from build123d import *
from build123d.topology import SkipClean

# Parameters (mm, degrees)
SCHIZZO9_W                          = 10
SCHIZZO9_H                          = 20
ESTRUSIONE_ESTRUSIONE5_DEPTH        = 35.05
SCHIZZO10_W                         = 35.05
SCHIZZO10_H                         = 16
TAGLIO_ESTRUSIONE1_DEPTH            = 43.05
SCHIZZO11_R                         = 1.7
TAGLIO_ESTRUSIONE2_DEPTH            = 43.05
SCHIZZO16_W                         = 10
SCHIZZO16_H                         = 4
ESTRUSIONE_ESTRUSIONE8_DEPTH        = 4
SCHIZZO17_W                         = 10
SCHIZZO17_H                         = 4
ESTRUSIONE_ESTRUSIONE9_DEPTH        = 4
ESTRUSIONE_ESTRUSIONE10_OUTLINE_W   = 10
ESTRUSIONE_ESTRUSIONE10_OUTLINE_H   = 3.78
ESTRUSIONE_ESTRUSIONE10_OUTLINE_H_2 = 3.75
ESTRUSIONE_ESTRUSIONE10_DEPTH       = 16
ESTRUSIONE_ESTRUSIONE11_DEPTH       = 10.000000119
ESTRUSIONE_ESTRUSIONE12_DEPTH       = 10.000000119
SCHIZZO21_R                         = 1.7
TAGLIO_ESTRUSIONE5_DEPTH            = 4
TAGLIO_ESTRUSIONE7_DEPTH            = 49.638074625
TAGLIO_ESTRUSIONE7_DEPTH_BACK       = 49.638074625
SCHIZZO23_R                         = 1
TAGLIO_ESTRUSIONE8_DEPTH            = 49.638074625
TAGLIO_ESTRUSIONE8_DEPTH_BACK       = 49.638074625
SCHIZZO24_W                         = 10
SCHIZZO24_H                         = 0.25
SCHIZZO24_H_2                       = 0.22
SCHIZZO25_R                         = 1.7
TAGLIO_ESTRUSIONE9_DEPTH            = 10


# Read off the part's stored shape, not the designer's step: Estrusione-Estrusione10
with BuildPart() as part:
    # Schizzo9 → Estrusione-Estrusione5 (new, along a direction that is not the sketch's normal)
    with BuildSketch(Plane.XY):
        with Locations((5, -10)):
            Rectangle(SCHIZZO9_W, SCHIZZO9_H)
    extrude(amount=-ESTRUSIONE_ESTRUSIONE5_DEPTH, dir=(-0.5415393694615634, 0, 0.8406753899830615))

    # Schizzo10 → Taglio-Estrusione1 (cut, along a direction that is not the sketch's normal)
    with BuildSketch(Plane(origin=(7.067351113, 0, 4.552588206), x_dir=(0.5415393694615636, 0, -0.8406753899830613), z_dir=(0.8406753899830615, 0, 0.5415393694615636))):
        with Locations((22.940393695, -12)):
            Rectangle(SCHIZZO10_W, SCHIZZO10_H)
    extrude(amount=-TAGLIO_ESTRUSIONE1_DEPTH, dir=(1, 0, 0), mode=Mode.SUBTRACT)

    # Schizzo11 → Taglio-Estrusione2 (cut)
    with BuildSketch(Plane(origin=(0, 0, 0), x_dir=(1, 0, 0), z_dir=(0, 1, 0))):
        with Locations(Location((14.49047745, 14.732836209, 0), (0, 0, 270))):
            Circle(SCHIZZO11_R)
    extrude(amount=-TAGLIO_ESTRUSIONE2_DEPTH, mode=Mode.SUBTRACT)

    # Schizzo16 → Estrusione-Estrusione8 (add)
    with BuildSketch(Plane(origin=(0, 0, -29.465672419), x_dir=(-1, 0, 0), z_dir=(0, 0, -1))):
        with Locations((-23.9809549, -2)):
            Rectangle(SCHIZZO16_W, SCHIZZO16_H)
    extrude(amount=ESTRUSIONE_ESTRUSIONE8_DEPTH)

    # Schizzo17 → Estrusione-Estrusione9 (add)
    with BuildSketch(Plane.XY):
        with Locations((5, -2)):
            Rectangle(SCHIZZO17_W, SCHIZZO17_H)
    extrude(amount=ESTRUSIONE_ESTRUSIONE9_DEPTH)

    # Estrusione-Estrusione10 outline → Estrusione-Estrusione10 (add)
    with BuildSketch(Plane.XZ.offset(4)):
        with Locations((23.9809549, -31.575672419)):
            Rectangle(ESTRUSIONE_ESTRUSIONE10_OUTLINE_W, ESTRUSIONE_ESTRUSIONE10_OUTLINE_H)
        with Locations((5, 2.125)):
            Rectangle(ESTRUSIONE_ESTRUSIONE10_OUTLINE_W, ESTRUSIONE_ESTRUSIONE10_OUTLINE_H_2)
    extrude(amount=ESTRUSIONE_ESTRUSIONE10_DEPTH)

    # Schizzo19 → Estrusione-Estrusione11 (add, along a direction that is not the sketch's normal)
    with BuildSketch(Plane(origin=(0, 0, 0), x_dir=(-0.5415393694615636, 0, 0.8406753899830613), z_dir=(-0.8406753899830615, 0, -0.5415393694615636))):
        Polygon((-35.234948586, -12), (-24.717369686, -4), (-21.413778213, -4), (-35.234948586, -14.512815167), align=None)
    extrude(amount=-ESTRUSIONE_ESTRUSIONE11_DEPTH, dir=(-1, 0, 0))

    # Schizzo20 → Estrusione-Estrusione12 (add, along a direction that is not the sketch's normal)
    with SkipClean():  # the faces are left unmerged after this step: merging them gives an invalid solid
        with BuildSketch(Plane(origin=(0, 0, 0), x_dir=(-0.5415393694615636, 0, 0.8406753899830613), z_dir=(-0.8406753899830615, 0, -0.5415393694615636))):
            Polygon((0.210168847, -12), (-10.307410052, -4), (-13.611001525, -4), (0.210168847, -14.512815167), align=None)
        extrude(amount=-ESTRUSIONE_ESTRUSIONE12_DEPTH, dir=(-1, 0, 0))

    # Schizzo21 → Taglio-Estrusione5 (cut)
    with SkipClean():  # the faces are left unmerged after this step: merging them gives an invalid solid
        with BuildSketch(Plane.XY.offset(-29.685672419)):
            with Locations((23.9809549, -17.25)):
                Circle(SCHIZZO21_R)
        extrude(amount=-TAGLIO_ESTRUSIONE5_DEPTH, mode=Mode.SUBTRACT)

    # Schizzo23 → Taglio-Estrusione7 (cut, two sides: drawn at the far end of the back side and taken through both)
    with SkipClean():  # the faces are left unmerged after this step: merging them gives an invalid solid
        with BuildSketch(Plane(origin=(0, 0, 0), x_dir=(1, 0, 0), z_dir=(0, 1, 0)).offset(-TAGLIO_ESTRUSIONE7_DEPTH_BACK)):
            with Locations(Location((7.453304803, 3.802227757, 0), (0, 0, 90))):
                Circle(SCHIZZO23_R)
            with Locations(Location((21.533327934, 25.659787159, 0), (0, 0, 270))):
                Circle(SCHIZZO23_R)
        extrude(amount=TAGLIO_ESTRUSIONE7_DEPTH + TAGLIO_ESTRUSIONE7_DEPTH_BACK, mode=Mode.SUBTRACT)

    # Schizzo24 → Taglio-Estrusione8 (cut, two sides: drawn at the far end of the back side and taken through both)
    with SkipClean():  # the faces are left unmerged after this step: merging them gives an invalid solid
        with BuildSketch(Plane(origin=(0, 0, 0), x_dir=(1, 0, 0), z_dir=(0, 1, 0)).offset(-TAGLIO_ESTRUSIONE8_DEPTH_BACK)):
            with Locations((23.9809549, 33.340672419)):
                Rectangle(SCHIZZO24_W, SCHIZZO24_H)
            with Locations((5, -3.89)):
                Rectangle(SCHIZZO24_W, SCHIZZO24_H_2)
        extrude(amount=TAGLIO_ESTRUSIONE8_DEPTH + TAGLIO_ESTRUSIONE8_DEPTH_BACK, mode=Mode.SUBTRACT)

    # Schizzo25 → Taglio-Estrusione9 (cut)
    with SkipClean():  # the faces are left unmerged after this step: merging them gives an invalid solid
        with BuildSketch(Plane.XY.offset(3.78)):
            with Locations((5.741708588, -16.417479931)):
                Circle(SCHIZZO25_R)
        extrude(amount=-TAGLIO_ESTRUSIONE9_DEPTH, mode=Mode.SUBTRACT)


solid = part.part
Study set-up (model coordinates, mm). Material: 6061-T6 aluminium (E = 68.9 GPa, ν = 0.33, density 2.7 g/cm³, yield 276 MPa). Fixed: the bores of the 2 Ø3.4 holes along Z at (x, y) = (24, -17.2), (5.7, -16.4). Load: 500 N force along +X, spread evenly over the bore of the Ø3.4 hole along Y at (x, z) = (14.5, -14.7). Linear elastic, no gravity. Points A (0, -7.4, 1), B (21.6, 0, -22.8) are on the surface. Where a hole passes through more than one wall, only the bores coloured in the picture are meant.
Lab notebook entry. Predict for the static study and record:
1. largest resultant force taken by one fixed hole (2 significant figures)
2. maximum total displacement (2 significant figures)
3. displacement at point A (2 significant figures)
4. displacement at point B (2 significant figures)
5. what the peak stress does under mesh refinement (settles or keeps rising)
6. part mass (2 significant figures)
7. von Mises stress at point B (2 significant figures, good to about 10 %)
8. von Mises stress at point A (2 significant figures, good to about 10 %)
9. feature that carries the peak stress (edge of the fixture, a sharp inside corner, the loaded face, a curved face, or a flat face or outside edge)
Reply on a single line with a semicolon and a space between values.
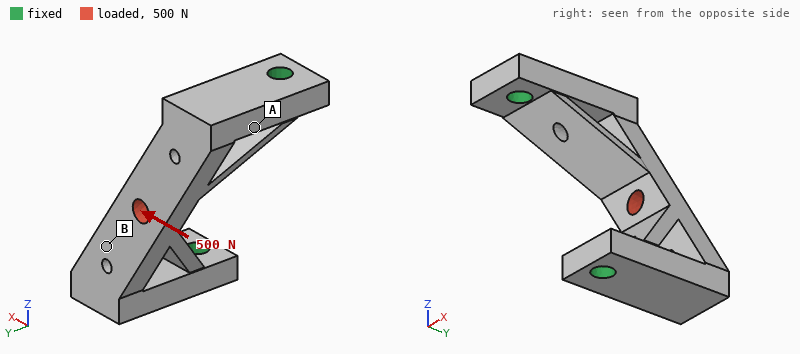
250 N; 69 µm; 21 µm; 56 µm; keeps rising; 8.1 g; 15 MPa; 34 MPa; edge of the fixture
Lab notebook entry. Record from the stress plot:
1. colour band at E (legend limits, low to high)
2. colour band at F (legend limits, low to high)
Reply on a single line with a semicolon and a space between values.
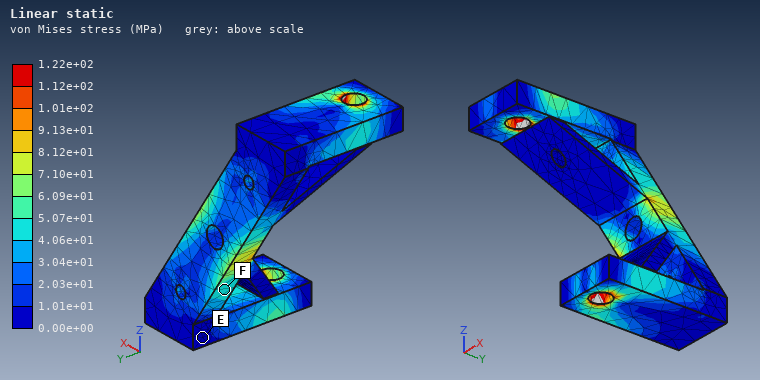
0.00e+00 to 1.01e+01 MPa; 4.06e+01 to 5.07e+01 MPa
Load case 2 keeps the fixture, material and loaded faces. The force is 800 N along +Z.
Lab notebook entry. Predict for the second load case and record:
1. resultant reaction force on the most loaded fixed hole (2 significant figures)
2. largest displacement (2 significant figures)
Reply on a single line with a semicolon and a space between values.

440 N; 0.10 mm
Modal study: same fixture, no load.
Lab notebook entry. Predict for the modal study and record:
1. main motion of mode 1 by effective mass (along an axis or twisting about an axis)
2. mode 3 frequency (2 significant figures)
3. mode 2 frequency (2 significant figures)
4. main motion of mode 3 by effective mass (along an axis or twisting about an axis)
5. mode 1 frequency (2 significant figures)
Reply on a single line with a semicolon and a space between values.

along Z; 7600 Hz; 6700 Hz; along X; 5700 Hz
